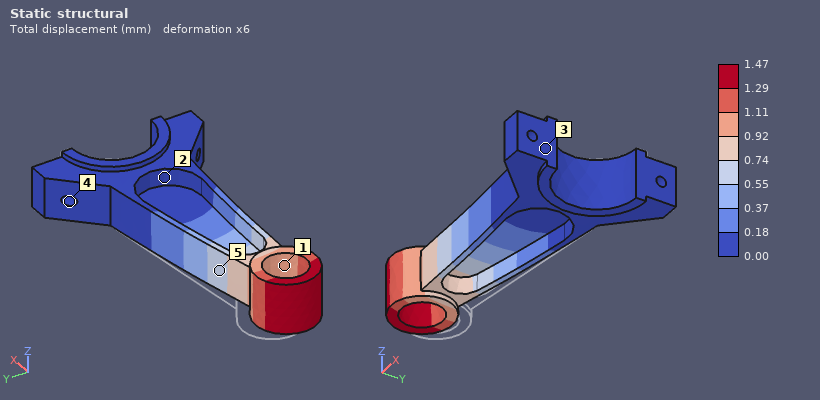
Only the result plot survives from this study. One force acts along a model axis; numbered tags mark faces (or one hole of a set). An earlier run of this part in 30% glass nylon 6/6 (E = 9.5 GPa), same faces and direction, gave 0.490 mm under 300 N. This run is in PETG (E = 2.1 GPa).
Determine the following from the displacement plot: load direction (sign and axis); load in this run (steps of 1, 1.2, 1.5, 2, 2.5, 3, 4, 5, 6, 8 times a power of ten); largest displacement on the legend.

-Y
200 N
1.47 mm
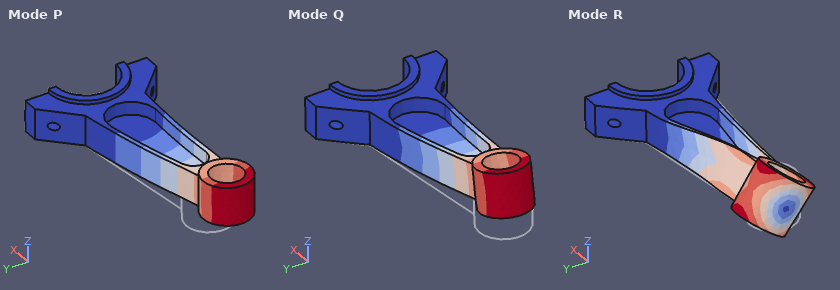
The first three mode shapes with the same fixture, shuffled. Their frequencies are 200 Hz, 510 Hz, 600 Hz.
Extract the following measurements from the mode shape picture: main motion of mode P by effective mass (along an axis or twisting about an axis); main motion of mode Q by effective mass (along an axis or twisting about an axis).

along Y
along Z
